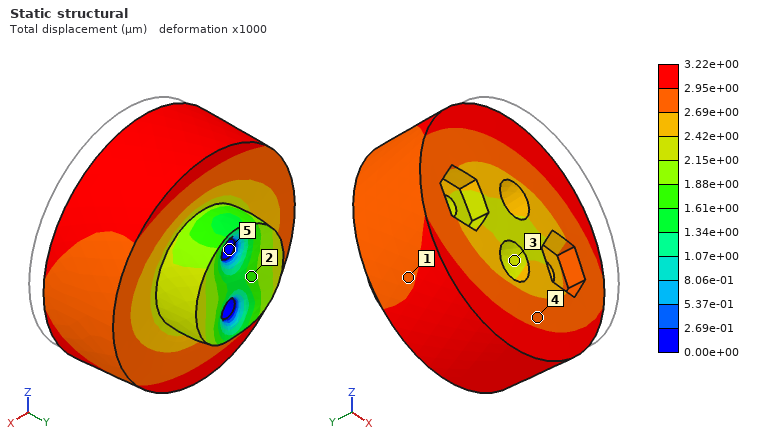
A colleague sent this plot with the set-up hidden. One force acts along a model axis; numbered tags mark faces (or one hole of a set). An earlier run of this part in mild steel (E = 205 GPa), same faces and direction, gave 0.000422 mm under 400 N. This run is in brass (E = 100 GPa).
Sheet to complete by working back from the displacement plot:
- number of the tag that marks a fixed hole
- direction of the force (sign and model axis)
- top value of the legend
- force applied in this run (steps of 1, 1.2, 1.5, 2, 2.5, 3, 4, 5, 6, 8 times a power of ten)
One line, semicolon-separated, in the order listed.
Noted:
5; +Y; 3.22e+00 µm; 1.5 kN
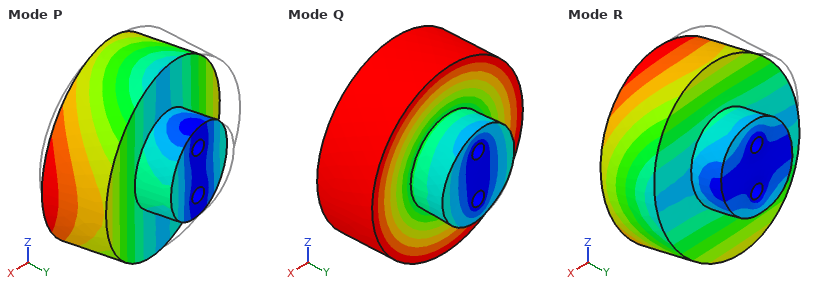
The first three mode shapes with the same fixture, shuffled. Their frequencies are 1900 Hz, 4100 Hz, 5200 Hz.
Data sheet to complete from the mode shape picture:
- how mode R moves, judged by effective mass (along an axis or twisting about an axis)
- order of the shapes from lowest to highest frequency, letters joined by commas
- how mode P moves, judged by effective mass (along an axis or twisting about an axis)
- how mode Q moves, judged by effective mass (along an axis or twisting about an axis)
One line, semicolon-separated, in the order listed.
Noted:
along Z; P, R, Q; along X; twisting about Y
